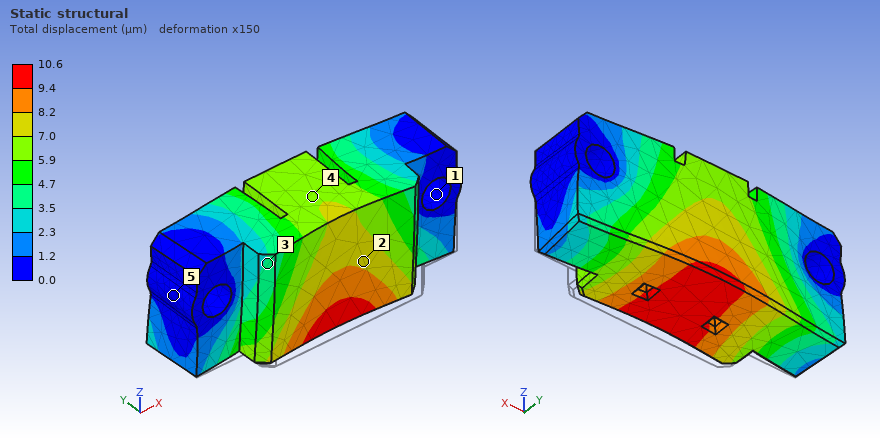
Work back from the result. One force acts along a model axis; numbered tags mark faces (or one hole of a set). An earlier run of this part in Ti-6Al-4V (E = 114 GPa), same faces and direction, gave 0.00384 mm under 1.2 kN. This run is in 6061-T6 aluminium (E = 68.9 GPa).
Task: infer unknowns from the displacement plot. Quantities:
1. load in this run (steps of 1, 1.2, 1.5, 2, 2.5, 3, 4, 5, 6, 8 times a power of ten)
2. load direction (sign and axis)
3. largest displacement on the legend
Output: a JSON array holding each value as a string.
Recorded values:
["2 kN", "+Y", "10.6 µm"]
